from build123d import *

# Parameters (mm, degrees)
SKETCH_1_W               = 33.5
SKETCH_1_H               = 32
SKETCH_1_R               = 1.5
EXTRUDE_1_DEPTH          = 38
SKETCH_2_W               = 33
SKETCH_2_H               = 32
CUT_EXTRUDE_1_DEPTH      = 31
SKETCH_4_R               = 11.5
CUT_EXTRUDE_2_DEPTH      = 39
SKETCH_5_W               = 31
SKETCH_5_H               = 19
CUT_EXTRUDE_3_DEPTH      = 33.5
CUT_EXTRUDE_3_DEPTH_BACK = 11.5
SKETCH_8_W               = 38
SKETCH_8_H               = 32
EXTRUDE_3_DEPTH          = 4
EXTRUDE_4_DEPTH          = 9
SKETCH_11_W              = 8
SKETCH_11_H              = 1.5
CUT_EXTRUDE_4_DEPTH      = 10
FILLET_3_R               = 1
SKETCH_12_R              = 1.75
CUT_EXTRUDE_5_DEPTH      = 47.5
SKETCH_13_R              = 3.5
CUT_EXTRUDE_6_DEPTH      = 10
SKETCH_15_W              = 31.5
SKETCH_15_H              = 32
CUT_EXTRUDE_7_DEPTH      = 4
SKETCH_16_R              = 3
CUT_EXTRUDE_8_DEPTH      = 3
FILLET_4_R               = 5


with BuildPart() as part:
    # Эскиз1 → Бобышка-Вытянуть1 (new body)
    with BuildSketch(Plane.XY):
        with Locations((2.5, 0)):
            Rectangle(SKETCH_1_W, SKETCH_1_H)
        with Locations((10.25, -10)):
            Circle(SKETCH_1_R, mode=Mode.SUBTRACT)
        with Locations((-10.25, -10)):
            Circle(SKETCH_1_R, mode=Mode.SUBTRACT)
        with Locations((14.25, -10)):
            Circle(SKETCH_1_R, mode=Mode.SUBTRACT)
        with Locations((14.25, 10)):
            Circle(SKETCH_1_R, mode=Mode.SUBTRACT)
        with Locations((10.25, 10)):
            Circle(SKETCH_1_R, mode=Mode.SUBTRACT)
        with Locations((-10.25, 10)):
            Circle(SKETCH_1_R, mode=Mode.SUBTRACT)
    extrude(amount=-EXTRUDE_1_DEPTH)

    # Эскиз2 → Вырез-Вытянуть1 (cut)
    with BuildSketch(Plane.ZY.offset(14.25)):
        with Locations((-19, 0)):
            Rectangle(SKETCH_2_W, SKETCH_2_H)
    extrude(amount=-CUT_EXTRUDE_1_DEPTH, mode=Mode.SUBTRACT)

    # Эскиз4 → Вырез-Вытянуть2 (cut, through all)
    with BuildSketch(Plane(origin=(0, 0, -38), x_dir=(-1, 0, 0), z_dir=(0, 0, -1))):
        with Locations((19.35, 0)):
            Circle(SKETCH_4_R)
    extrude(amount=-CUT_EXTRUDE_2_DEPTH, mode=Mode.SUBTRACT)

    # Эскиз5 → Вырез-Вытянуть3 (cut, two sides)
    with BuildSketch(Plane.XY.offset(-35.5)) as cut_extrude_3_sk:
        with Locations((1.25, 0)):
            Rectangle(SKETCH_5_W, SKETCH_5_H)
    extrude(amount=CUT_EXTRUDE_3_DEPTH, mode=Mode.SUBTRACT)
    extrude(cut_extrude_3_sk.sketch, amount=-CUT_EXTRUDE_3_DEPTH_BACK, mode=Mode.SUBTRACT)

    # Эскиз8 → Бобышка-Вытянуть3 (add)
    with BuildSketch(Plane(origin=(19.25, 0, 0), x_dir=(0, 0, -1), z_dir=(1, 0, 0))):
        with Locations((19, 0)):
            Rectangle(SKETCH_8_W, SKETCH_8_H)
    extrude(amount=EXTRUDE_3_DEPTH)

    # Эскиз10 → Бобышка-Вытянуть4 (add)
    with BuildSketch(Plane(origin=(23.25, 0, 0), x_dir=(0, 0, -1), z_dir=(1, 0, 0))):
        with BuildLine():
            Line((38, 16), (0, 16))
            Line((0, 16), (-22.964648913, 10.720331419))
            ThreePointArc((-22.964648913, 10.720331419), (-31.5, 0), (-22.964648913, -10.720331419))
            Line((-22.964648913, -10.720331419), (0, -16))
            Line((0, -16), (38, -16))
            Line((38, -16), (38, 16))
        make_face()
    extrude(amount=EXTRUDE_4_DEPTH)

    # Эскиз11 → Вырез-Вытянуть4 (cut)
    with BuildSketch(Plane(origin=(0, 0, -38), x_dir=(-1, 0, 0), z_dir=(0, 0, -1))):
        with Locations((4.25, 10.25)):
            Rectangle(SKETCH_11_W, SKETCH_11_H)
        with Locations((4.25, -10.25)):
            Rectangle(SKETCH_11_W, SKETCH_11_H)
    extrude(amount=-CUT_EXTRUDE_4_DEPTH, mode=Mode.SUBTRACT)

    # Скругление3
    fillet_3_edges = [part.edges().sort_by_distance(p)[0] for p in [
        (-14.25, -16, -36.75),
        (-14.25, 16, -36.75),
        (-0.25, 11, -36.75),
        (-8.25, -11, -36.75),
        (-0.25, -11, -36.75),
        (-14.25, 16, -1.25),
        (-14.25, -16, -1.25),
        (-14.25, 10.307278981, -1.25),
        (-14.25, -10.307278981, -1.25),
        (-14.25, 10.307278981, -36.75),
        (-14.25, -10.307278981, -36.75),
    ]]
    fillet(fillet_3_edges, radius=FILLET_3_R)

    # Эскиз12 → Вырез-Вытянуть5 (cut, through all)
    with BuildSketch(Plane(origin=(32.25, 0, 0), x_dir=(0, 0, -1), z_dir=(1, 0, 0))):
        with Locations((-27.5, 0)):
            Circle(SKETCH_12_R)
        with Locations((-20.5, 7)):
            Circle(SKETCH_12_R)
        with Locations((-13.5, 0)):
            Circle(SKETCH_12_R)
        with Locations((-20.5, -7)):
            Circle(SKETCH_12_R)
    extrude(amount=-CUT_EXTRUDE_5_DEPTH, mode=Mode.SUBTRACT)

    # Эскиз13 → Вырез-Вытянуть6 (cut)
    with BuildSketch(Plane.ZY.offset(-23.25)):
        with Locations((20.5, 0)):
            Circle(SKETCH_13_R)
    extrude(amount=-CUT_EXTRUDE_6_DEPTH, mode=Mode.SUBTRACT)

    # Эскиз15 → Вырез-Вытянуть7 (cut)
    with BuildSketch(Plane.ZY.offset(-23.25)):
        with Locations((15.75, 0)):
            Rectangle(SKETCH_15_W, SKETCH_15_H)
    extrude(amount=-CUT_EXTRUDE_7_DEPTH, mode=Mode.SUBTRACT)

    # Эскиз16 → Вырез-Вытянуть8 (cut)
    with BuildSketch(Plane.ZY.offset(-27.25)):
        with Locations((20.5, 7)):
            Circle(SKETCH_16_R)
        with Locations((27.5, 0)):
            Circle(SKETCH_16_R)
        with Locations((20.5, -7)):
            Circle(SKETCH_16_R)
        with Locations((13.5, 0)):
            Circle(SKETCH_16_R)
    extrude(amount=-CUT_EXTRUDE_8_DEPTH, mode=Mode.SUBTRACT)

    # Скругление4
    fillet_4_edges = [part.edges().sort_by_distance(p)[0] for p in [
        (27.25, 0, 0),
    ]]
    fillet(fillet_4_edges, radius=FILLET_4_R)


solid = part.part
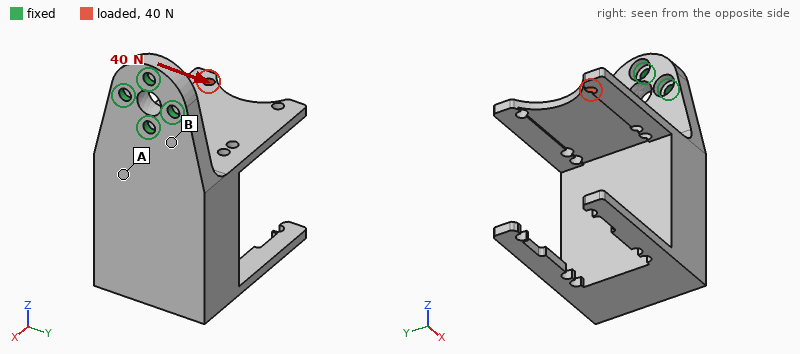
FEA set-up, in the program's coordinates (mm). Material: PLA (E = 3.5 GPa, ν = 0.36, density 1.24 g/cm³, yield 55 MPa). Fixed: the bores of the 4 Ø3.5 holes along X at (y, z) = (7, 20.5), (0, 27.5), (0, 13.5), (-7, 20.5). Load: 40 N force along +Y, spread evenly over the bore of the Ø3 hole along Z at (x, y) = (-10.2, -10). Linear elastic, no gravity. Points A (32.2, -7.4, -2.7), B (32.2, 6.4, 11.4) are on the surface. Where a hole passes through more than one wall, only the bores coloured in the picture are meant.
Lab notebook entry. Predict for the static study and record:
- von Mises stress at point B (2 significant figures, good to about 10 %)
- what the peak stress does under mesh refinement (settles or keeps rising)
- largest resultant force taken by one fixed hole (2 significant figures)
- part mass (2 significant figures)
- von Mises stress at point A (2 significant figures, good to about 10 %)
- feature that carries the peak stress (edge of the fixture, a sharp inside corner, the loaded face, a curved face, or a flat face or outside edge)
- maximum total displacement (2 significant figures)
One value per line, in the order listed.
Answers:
7.5 MPa
keeps rising
97 N
31 g
3.3 MPa
edge of the fixture
0.90 mm
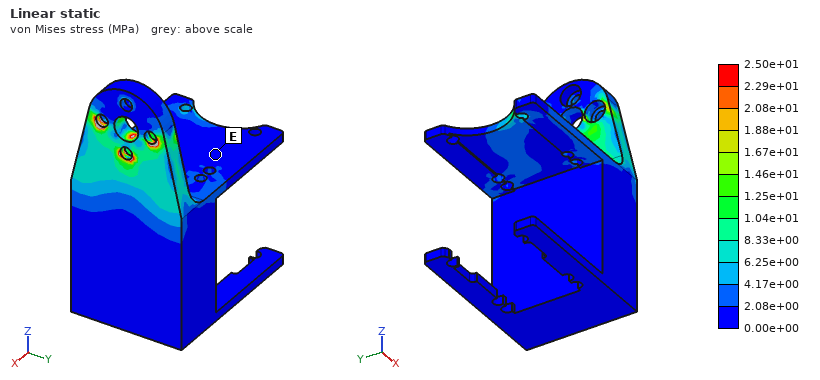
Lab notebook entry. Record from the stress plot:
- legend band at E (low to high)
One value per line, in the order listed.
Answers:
0.00e+00 to 2.08e+00 MPa
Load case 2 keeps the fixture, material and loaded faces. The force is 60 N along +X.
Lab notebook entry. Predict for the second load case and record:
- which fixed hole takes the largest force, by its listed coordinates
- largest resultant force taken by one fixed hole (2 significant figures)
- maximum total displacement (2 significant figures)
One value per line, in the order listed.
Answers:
(0, 13.5)
150 N
0.86 mm
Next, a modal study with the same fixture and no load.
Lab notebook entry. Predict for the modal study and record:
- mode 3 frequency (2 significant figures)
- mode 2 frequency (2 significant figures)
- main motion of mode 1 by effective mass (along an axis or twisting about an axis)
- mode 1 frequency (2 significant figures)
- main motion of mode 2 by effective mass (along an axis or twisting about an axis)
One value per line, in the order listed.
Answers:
630 Hz
570 Hz
along X
220 Hz
along Y
